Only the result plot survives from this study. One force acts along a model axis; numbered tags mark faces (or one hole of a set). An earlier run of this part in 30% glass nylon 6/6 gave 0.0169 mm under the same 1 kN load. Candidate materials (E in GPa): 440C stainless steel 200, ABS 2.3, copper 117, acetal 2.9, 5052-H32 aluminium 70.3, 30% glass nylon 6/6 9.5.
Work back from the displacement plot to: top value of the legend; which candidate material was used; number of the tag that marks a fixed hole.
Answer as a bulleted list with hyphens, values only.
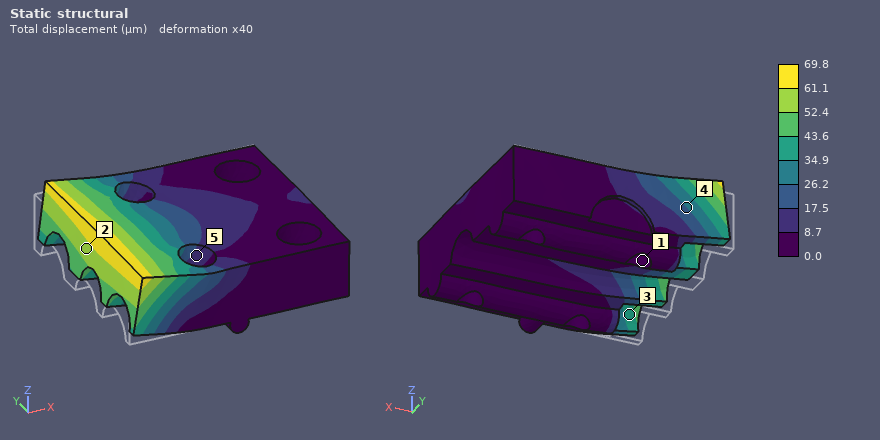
- 69.8 µm
- ABS
- 1
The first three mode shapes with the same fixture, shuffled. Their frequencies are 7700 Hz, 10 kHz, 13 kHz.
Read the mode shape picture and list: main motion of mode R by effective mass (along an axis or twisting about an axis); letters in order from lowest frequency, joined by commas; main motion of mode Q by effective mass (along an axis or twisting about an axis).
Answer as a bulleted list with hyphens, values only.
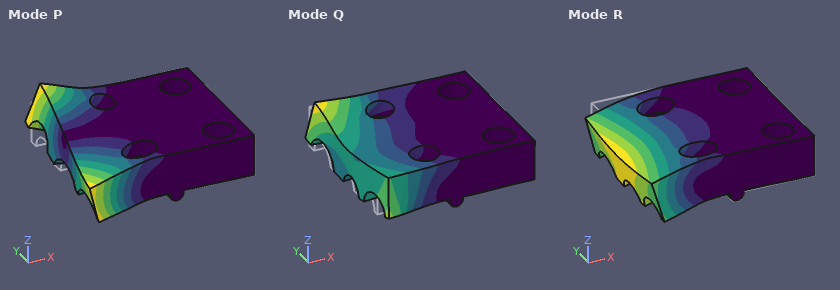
- along Z
- R, P, Q
- along Y
